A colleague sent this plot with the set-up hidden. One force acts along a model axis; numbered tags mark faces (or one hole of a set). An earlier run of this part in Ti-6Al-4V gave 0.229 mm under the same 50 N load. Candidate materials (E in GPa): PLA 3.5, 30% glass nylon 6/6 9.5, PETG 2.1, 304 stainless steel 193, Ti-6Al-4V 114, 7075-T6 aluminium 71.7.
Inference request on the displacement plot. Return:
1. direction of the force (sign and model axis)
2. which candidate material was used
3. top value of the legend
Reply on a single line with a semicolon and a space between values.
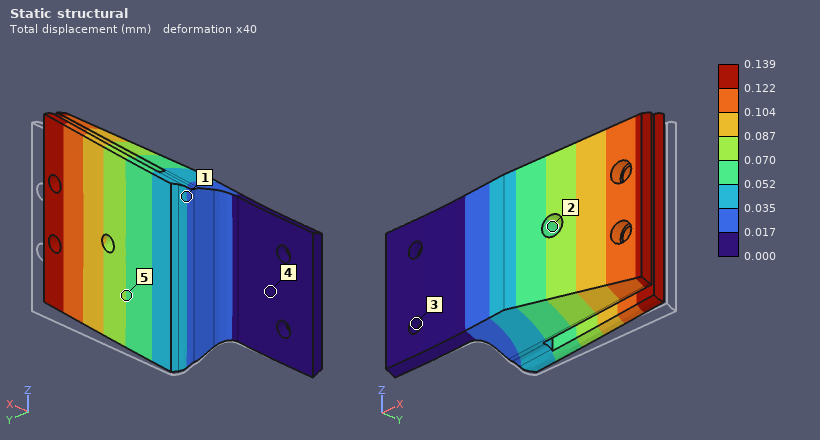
-Y; 304 stainless steel; 0.139 mm
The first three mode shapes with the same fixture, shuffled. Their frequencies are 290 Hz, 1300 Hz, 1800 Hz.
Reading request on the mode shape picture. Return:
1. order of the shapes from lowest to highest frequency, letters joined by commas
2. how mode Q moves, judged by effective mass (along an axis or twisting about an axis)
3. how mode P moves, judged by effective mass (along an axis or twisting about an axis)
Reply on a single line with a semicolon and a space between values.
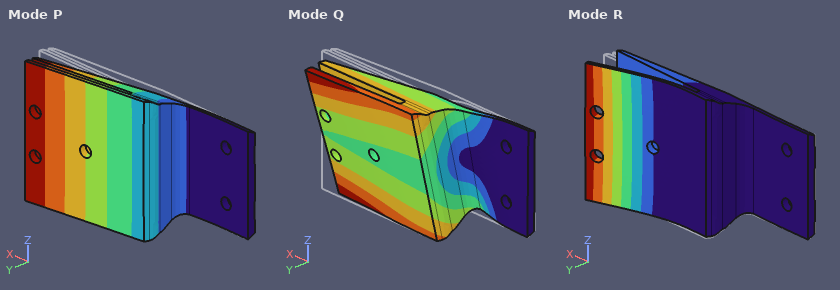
P, Q, R; along Z; along Y
